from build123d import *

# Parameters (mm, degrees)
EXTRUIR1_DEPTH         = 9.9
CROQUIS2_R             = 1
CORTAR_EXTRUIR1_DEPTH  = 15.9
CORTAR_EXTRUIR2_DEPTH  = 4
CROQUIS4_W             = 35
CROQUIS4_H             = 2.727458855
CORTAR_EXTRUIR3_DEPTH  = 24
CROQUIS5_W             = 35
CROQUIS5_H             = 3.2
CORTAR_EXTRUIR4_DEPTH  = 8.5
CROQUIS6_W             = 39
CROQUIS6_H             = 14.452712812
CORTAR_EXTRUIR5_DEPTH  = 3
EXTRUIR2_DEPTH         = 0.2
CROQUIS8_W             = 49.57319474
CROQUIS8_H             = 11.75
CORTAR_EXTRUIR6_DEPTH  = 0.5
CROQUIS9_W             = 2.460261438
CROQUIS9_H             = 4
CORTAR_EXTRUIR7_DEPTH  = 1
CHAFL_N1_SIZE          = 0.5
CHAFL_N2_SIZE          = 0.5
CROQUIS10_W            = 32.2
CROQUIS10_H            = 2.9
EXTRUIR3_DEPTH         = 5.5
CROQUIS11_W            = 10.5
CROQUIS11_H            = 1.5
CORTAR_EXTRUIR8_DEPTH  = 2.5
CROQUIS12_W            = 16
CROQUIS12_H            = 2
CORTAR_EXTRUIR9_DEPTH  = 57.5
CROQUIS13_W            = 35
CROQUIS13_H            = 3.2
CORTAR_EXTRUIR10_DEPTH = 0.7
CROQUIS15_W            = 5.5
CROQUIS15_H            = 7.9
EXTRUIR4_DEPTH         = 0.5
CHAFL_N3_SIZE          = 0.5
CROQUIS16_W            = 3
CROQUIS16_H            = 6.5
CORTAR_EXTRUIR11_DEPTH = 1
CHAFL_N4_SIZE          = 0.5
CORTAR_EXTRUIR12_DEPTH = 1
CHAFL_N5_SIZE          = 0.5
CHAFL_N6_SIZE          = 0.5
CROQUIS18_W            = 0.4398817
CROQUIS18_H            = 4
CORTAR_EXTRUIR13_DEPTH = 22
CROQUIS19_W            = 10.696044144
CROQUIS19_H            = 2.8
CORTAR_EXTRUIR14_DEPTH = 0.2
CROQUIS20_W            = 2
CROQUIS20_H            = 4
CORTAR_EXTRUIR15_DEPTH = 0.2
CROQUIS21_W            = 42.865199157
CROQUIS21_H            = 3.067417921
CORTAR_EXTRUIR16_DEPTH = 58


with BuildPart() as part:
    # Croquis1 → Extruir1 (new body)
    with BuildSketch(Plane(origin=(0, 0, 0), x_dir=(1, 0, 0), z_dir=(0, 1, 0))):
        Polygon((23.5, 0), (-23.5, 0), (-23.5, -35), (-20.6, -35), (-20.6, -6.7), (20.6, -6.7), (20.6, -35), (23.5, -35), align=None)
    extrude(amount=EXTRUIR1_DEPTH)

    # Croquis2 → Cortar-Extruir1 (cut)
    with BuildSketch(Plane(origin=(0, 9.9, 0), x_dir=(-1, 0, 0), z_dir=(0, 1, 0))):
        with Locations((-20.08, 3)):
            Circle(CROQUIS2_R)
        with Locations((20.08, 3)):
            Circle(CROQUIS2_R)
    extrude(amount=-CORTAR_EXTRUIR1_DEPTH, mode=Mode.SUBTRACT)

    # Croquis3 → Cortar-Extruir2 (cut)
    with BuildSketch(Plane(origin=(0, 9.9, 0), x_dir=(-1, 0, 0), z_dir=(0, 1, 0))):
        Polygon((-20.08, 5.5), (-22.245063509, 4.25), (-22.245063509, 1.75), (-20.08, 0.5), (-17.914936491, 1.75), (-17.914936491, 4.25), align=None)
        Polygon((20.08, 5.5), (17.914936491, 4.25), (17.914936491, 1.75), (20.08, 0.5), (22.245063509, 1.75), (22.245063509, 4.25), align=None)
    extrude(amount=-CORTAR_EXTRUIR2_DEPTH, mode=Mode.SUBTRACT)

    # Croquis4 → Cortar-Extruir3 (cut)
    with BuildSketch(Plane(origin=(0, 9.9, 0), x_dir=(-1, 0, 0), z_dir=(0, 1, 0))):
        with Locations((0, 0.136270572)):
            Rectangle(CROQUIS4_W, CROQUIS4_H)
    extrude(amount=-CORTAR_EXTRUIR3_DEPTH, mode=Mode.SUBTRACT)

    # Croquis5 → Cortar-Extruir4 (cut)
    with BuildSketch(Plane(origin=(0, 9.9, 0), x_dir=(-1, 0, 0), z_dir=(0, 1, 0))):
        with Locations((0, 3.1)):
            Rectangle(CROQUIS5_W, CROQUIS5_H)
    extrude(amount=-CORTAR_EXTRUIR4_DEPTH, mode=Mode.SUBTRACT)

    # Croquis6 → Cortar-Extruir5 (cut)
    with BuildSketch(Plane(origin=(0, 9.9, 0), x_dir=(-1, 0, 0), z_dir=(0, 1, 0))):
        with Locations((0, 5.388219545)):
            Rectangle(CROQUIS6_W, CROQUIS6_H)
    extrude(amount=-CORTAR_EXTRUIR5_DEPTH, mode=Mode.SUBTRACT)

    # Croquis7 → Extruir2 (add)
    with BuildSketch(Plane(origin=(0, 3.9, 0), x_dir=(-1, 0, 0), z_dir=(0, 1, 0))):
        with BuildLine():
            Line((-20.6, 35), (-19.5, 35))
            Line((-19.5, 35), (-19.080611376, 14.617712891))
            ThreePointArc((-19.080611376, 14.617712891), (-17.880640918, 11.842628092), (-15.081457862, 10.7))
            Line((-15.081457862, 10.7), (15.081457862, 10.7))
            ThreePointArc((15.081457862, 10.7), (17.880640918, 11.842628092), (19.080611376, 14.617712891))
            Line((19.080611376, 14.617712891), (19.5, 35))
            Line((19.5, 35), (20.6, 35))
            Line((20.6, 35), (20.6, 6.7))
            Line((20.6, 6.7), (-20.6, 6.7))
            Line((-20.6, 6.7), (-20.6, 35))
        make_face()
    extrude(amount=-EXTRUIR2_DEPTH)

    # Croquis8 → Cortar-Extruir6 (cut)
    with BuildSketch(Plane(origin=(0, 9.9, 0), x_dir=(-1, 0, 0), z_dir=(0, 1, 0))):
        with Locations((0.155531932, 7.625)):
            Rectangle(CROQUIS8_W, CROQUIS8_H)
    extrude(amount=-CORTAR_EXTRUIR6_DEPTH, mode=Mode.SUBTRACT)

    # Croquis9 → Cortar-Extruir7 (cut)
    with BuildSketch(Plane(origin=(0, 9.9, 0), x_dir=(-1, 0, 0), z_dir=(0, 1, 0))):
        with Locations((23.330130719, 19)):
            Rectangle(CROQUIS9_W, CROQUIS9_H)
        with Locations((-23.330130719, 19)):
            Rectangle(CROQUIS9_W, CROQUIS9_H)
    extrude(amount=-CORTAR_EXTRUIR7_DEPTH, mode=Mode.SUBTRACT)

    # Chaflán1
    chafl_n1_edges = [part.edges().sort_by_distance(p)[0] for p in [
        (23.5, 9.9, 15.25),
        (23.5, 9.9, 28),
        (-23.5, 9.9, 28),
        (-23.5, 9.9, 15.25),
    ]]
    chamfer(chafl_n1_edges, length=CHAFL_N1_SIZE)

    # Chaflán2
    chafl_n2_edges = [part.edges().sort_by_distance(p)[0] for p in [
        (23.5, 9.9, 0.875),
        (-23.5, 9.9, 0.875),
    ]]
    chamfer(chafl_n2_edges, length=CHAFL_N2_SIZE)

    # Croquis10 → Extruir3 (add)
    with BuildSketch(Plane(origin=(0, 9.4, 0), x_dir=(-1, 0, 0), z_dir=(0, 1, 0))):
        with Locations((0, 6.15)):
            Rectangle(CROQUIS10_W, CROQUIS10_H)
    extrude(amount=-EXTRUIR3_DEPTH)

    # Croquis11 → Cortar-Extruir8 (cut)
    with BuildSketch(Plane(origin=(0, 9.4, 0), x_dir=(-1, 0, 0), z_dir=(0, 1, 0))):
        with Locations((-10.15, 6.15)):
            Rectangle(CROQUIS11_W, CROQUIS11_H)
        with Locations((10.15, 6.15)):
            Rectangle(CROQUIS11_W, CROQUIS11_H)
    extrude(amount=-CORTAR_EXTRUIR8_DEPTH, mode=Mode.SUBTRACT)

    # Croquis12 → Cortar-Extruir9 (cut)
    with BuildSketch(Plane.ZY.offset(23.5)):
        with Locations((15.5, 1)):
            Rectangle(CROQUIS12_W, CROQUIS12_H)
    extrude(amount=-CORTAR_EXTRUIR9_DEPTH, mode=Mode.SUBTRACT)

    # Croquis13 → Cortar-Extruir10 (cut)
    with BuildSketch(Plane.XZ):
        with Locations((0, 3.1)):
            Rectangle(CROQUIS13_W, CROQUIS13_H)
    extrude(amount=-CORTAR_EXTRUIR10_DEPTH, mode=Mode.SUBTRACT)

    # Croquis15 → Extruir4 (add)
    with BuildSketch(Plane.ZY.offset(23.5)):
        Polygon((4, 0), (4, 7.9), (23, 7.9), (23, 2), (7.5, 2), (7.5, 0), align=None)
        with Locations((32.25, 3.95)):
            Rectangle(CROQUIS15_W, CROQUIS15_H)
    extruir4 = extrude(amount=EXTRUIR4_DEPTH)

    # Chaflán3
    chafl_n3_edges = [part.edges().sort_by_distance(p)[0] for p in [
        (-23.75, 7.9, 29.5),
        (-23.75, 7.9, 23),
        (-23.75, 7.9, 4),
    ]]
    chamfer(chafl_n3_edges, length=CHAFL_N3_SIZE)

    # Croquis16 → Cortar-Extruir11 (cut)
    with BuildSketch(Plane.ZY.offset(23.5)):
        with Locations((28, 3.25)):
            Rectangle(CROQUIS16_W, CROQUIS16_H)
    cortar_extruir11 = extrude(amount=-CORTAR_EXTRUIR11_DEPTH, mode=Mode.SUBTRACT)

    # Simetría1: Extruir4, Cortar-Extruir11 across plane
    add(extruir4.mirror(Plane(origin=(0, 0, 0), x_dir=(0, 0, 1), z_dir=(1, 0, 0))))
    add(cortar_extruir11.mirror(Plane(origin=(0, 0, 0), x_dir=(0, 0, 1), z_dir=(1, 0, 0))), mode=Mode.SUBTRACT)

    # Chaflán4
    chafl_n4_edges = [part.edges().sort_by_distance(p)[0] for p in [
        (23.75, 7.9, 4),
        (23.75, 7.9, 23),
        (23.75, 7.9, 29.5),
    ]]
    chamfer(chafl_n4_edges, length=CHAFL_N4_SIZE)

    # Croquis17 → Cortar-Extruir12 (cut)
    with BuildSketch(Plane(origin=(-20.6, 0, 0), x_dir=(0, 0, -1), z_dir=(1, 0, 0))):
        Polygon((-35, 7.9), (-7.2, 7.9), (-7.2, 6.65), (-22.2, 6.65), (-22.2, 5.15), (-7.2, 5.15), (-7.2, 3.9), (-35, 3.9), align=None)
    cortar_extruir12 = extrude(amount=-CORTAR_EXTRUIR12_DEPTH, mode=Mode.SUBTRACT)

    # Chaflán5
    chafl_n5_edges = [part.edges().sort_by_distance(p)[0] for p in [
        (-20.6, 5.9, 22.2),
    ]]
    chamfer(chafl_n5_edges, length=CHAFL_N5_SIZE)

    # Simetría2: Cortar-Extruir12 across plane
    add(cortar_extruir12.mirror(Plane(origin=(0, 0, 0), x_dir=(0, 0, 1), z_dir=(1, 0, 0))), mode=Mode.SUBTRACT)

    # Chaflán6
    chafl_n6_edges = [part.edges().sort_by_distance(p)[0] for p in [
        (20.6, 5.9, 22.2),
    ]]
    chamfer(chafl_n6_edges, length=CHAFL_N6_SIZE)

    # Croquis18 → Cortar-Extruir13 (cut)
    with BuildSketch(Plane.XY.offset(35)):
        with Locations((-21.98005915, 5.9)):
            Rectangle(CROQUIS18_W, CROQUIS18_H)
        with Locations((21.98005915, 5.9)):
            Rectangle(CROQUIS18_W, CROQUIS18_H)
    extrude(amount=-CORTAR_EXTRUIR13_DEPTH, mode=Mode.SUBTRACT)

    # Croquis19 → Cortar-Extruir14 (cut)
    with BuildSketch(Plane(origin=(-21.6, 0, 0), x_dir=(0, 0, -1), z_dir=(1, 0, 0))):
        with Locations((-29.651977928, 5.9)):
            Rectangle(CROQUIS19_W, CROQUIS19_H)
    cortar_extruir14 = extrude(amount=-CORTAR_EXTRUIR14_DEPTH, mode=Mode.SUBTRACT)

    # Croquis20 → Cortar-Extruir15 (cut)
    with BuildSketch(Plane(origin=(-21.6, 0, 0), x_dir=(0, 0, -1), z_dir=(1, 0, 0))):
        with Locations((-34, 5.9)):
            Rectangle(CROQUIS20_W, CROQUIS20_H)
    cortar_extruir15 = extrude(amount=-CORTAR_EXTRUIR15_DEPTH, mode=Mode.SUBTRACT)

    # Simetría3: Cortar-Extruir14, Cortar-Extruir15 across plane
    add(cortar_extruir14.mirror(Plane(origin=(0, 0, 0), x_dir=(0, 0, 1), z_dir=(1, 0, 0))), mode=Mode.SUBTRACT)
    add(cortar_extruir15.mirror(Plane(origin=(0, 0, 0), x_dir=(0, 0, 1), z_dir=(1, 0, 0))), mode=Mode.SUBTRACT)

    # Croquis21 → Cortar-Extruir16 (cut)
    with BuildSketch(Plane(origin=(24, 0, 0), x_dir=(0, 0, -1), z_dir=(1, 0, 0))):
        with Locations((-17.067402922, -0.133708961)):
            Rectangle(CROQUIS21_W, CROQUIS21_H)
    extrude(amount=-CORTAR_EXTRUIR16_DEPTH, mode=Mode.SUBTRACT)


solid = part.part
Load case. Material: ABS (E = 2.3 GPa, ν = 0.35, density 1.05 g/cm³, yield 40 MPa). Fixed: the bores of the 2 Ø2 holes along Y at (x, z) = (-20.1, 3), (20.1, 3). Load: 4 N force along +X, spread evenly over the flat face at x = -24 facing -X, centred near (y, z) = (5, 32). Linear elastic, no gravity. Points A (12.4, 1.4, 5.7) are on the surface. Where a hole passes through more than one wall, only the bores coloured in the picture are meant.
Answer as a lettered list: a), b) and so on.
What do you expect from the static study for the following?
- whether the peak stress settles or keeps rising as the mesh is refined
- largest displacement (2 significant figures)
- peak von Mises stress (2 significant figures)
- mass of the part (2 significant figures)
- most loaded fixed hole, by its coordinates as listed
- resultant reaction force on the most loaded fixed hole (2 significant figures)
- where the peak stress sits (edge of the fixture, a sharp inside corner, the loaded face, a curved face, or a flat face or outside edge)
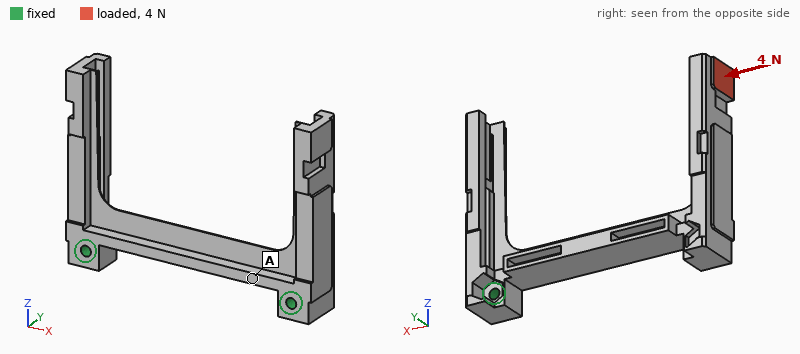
a) settles
b) 0.64 mm
c) 26 MPa
d) 2.4 g
e) (20.1, 3)
f) 5.6 N
g) a curved face
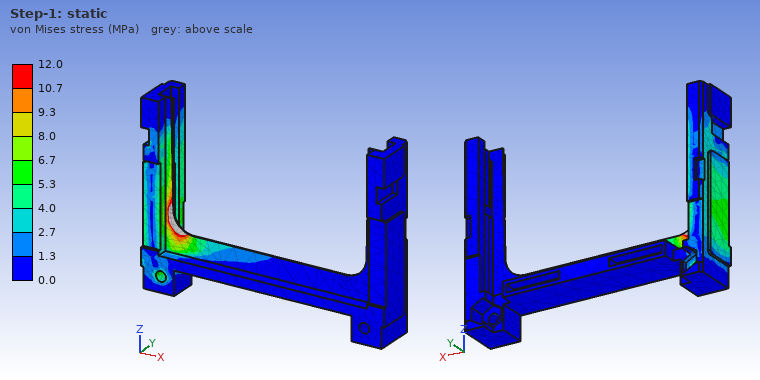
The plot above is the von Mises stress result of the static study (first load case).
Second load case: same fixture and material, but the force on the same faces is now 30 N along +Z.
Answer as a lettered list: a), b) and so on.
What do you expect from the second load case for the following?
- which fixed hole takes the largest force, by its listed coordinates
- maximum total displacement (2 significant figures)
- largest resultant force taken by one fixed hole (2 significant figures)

a) (-20.1, 3)
b) 0.62 mm
c) 31 N
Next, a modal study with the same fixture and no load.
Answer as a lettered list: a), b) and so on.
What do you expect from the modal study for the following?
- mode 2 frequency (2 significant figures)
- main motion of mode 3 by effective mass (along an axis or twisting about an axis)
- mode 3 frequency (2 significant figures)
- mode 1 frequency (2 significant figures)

a) 980 Hz
b) along Y
c) 1400 Hz
d) 970 Hz
